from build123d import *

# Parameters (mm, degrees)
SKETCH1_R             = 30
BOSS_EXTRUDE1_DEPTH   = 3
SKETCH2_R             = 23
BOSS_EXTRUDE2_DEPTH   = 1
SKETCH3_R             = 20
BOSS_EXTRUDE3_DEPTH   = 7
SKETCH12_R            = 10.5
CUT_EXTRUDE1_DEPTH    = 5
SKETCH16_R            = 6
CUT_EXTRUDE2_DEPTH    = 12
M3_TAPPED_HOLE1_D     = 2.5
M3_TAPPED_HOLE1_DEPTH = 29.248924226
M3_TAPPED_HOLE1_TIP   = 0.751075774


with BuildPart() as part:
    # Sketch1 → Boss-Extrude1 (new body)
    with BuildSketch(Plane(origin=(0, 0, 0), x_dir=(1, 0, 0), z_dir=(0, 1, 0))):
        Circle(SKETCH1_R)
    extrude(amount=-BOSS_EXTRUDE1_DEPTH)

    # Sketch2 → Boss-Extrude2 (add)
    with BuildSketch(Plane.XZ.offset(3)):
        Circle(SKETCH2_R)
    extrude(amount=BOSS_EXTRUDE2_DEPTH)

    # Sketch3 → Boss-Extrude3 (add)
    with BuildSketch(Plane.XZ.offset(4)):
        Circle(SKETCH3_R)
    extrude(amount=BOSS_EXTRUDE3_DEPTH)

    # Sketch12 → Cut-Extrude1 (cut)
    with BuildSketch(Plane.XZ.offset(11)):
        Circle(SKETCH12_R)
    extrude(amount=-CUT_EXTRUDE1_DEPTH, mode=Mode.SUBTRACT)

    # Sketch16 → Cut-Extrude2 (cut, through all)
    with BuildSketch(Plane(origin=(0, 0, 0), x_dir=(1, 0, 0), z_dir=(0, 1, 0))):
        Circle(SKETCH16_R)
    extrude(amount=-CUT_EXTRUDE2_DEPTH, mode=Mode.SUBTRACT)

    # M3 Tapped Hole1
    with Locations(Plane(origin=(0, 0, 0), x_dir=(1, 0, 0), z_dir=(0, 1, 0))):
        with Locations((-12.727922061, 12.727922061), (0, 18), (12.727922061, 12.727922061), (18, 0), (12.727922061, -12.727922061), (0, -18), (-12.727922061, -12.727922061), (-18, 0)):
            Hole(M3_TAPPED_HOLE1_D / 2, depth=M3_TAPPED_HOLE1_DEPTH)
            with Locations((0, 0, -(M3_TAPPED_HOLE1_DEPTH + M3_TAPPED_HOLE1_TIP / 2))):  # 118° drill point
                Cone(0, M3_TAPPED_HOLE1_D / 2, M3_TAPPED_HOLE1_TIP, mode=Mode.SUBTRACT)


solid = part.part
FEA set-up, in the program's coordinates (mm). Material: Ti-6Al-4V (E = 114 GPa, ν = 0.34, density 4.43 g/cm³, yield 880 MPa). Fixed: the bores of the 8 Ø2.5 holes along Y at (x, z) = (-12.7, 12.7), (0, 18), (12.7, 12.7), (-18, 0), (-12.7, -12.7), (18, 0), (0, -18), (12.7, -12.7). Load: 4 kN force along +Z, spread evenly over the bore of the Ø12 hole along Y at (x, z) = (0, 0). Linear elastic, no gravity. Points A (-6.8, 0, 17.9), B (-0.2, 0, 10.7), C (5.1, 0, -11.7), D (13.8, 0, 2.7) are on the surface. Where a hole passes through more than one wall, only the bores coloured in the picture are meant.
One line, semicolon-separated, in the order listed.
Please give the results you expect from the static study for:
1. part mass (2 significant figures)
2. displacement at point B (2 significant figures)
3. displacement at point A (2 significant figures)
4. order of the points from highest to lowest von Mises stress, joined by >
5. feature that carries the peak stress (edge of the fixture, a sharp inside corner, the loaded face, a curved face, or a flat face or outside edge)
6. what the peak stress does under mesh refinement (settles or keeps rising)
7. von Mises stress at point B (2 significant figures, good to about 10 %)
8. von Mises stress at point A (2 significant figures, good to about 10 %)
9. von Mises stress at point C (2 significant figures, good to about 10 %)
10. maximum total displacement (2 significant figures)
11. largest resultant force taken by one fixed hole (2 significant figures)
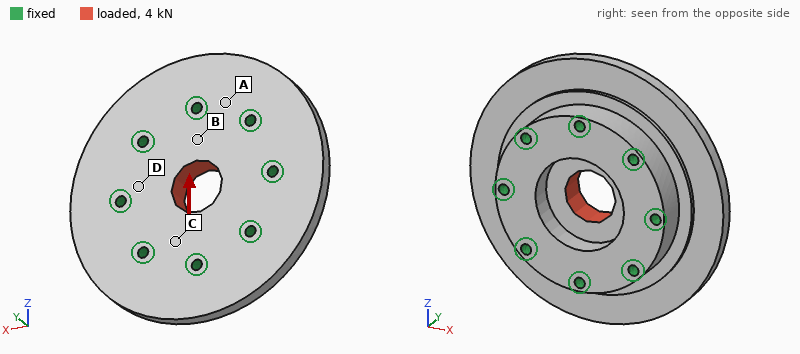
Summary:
71 g; 1.1 µm; 0.43 µm; B > C > A > D; edge of the fixture; keeps rising; 16 MPa; 4.9 MPa; 8.9 MPa; 1.8 µm; 820 N
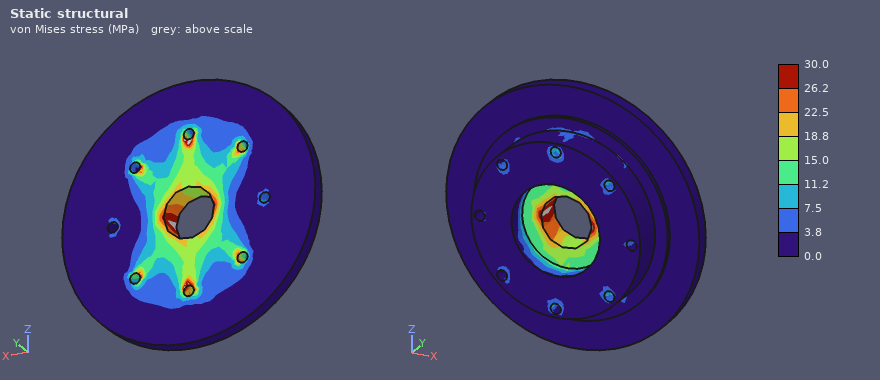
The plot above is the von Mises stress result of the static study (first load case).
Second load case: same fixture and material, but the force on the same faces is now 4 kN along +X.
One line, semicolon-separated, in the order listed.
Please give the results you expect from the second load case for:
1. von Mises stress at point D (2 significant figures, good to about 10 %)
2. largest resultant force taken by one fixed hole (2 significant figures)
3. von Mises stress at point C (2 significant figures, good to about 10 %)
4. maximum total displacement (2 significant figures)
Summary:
12 MPa; 820 N; 5.1 MPa; 1.9 µm
